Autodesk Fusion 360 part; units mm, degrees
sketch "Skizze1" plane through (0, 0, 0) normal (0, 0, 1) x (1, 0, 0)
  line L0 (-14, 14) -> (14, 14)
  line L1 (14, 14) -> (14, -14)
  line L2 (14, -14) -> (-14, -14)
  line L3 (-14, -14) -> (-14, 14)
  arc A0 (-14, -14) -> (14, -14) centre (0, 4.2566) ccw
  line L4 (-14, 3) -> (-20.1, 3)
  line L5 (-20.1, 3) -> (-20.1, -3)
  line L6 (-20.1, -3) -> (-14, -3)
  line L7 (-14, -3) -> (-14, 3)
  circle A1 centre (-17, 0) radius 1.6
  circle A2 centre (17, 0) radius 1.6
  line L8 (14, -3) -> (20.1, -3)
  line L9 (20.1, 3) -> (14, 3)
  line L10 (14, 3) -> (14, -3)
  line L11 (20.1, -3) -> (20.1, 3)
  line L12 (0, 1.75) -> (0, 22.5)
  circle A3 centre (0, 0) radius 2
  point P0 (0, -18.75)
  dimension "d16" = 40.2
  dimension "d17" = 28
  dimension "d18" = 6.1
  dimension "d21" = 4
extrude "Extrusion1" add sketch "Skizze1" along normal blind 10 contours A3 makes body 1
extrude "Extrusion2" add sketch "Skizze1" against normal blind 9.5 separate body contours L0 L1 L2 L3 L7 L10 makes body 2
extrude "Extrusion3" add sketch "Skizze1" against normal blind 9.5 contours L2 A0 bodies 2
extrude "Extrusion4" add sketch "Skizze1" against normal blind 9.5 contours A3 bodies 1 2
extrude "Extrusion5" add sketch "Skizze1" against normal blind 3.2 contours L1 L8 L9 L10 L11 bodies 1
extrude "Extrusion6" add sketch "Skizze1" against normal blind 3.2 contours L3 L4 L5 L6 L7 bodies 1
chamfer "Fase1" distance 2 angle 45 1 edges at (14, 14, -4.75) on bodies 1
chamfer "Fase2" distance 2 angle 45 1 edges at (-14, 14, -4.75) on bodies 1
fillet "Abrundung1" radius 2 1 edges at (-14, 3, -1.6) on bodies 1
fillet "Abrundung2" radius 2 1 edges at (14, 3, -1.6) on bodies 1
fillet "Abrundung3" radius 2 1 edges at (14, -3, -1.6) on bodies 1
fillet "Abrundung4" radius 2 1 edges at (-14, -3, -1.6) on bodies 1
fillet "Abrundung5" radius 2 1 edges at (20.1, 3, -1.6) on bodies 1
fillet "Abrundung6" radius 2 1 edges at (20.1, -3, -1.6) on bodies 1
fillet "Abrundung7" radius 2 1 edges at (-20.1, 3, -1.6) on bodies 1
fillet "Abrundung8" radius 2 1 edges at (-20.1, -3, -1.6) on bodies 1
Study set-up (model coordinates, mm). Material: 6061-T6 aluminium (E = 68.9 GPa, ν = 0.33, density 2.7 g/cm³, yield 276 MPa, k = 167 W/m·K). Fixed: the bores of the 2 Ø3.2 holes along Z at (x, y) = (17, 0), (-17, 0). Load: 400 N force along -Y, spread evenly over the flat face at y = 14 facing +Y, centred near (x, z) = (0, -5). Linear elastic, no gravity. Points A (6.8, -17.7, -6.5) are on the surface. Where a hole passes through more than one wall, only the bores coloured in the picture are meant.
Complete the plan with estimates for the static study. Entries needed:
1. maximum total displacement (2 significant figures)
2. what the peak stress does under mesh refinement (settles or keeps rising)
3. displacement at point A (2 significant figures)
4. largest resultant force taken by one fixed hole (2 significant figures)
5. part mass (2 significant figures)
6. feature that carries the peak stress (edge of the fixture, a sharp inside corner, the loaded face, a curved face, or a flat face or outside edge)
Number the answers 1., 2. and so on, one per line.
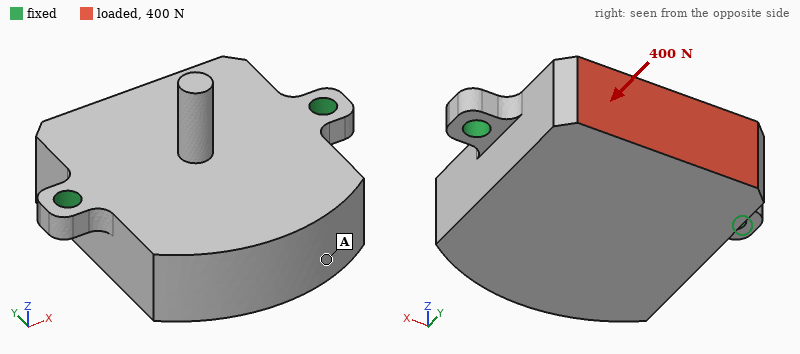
1. 24 µm
2. keeps rising
3. 21 µm
4. 200 N
5. 23 g
6. edge of the fixture
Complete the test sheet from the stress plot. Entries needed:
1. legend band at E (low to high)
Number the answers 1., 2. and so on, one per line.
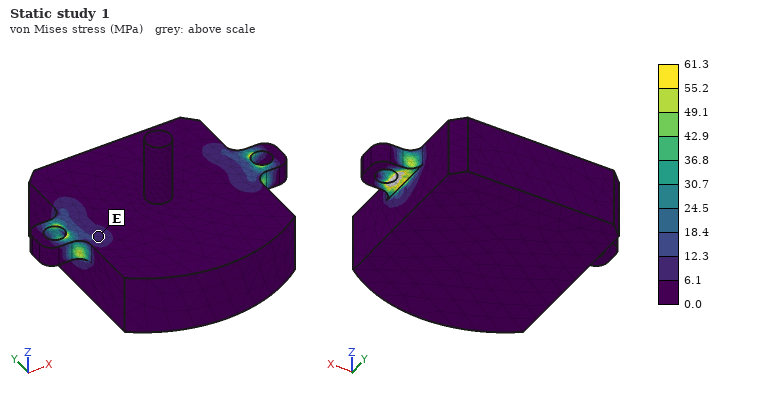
1. 6.1 to 12.3 MPa
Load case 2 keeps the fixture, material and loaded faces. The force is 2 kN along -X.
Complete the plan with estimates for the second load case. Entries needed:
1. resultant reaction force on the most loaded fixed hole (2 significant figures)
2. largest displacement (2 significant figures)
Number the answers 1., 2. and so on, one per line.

1. 1.3 kN
2. 15 µm
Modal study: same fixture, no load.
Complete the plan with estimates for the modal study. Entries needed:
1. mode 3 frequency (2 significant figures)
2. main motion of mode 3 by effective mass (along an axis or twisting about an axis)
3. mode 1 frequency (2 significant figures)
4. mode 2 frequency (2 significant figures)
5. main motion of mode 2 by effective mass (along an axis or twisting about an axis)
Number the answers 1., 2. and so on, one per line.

1. 18 kHz
2. along Y
3. 3500 Hz
4. 12 kHz
5. along Z
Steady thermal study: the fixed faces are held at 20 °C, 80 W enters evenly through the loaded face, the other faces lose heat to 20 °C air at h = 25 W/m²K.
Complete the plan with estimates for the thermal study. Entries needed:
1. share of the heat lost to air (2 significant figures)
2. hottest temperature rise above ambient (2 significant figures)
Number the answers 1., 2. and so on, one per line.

1. 3.9 %
2. 69 K
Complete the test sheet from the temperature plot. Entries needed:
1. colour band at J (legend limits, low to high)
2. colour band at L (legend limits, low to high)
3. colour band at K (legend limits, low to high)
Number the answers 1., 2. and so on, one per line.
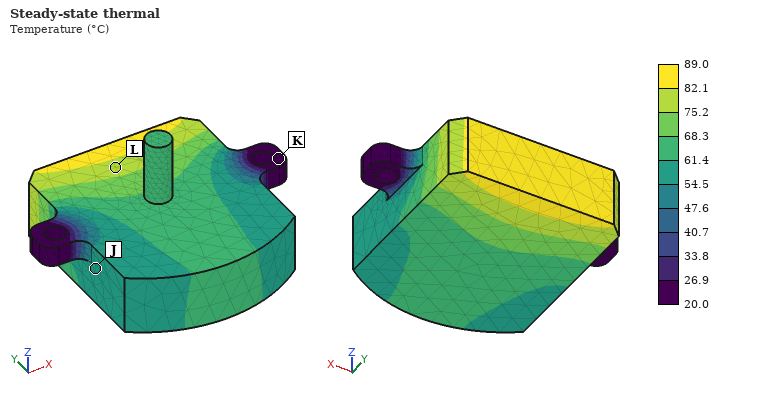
1. 54.5 to 61.4 °C
2. 75.2 to 82.1 °C
3. 20.0 to 26.9 °C
